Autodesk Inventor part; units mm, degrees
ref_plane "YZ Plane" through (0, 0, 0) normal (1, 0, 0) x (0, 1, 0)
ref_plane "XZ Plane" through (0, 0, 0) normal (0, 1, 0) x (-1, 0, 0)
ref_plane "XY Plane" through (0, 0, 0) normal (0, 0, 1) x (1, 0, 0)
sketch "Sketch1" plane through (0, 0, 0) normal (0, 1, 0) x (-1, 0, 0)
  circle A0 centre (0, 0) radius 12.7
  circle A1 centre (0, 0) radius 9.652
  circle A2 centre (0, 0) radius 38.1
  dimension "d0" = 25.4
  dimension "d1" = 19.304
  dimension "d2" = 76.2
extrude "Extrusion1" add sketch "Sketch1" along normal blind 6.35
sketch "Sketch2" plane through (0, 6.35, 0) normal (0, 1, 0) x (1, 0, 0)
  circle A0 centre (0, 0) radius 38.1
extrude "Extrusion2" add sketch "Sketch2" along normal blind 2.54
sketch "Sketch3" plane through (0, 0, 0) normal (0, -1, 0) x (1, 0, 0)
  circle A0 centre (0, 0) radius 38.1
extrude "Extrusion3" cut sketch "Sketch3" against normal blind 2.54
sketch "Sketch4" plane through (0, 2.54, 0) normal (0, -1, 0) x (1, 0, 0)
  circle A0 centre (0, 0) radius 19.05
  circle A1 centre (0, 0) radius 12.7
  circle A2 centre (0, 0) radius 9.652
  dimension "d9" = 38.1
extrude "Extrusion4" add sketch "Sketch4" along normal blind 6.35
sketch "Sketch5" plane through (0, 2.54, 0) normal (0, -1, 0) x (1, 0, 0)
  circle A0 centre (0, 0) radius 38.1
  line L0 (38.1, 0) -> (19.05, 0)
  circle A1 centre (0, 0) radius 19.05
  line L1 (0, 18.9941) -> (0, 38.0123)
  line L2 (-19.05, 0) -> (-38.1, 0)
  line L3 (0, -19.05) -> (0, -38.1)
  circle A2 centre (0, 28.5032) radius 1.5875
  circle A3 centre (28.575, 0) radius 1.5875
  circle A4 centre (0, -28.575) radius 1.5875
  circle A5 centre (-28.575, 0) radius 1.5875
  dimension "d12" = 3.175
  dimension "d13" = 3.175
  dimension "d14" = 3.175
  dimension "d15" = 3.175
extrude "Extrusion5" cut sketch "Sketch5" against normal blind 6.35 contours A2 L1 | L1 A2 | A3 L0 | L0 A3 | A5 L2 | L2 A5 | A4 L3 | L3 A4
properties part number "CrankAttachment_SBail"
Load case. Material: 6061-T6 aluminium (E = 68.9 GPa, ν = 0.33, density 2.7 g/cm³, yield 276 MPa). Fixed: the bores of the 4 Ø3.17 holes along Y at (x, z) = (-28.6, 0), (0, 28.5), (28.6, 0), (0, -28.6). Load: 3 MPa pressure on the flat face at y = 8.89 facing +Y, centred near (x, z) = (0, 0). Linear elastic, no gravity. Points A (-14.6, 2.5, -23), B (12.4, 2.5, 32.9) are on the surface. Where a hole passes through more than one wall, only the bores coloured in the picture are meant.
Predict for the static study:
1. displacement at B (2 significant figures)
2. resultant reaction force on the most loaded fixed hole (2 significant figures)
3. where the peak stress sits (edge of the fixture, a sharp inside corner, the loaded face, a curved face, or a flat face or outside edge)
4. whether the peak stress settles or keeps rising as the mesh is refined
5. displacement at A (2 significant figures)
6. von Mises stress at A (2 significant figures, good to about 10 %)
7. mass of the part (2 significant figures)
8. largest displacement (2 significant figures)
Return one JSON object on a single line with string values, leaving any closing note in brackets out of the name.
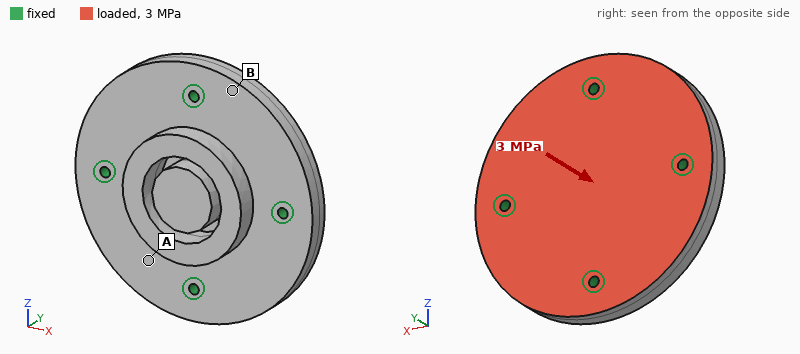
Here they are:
{"displacement at B": "20 µm", "resultant reaction force on the most loaded fixed hole": "3.4 kN", "where the peak stress sits": "edge of the fixture", "whether the peak stress settles or keeps rising as the mesh is refined": "keeps rising", "displacement at A": "25 µm", "von Mises stress at A": "30 MPa", "mass of the part": "91 g", "largest displacement": "41 µm"}
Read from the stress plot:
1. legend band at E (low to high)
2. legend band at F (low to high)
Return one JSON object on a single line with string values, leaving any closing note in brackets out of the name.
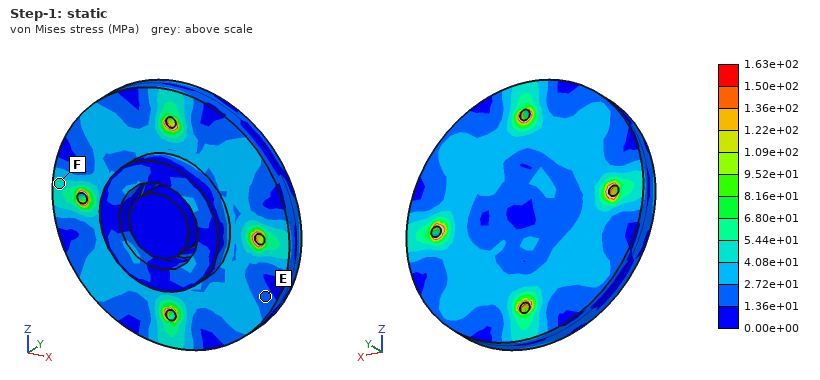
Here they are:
{"legend band at E": "1.36e+01 to 2.72e+01 MPa", "legend band at F": "4.08e+01 to 5.44e+01 MPa"}
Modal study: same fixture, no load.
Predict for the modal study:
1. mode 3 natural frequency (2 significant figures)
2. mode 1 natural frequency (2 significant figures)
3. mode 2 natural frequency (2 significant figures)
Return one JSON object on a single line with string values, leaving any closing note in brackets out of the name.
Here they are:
{"mode 3 natural frequency": "12 kHz", "mode 1 natural frequency": "11 kHz", "mode 2 natural frequency": "12 kHz"}
